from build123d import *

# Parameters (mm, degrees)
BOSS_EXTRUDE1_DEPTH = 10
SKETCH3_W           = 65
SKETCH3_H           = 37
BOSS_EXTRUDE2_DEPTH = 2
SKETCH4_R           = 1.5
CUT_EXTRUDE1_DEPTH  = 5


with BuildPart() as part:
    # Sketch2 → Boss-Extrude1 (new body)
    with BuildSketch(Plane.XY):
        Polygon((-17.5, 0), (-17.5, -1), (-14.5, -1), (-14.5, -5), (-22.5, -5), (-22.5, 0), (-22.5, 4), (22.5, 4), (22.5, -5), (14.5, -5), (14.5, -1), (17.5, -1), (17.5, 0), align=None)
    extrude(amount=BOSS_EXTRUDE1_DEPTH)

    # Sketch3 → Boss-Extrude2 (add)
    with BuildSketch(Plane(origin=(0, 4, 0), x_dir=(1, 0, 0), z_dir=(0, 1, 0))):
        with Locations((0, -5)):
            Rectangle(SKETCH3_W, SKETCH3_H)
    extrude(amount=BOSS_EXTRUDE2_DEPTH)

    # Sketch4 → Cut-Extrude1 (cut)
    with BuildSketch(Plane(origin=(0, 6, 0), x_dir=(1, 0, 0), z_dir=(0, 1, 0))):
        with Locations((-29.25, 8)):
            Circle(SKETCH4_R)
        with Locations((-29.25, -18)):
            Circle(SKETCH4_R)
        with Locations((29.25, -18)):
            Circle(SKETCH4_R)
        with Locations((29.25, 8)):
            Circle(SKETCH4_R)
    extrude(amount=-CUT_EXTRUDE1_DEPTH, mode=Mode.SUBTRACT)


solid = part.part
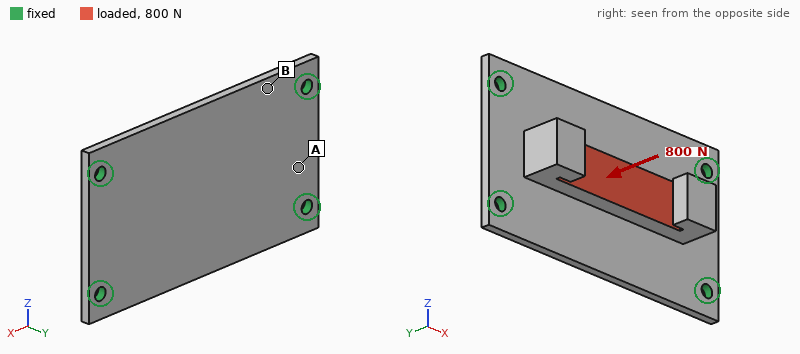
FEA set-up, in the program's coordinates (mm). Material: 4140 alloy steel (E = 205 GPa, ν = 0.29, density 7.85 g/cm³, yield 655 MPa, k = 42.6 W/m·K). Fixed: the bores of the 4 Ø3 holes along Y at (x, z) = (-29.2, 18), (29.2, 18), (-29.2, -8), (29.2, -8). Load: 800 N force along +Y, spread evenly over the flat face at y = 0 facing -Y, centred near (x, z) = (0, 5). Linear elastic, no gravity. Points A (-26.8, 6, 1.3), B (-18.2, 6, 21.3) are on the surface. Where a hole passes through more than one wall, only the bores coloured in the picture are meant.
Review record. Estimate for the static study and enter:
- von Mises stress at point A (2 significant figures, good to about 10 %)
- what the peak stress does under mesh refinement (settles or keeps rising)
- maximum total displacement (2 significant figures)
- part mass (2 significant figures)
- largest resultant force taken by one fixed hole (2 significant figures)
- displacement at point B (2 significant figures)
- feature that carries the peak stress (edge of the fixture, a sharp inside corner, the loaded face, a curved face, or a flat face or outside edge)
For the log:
44 MPa
keeps rising
40 µm
57 g
350 N
15 µm
edge of the fixture
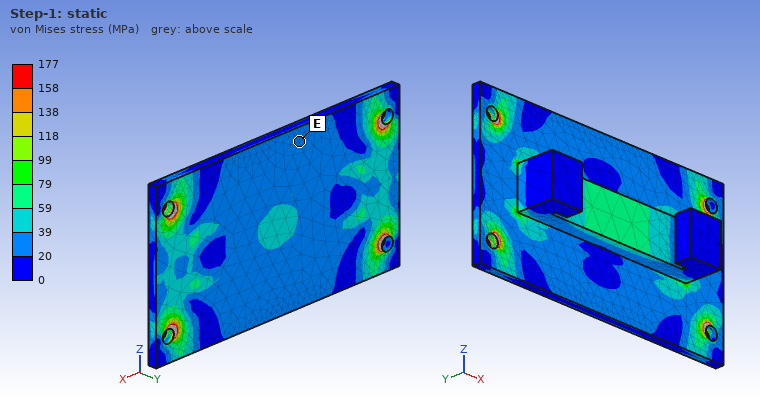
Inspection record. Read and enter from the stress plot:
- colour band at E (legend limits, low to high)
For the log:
20 to 39 MPa
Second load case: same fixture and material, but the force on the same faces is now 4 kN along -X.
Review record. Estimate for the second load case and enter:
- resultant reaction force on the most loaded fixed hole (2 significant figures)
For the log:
1.1 kN
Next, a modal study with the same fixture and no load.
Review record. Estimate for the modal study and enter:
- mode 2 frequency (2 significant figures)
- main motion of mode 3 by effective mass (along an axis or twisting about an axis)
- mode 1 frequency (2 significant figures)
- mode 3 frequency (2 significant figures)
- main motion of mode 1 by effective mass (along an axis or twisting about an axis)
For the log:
5600 Hz
twisting about Z
3900 Hz
8500 Hz
along Y
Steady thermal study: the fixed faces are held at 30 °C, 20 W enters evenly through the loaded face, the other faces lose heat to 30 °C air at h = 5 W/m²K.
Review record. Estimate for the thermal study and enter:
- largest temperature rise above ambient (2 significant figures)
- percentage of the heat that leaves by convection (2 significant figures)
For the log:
72 K
5.8 %
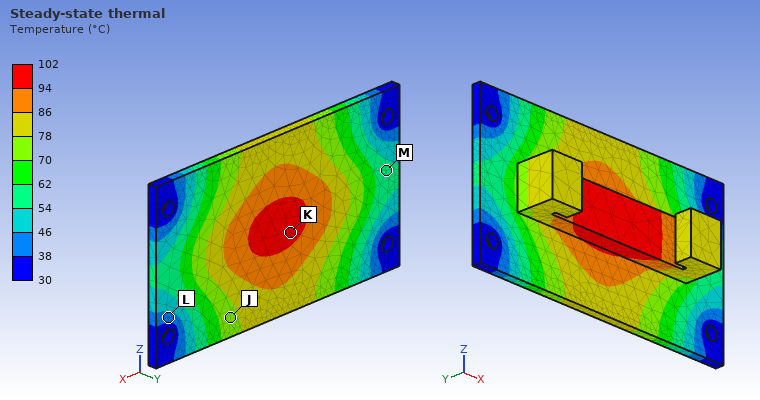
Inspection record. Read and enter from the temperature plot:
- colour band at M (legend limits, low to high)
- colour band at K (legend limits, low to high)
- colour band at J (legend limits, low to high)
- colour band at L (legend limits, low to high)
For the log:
54 to 62 °C
94 to 102 °C
70 to 78 °C
38 to 46 °C
